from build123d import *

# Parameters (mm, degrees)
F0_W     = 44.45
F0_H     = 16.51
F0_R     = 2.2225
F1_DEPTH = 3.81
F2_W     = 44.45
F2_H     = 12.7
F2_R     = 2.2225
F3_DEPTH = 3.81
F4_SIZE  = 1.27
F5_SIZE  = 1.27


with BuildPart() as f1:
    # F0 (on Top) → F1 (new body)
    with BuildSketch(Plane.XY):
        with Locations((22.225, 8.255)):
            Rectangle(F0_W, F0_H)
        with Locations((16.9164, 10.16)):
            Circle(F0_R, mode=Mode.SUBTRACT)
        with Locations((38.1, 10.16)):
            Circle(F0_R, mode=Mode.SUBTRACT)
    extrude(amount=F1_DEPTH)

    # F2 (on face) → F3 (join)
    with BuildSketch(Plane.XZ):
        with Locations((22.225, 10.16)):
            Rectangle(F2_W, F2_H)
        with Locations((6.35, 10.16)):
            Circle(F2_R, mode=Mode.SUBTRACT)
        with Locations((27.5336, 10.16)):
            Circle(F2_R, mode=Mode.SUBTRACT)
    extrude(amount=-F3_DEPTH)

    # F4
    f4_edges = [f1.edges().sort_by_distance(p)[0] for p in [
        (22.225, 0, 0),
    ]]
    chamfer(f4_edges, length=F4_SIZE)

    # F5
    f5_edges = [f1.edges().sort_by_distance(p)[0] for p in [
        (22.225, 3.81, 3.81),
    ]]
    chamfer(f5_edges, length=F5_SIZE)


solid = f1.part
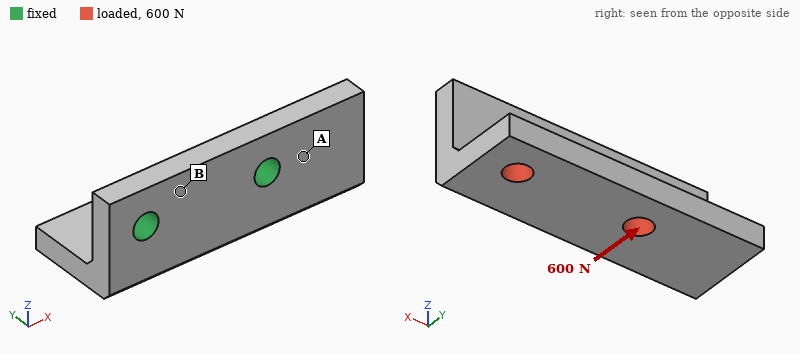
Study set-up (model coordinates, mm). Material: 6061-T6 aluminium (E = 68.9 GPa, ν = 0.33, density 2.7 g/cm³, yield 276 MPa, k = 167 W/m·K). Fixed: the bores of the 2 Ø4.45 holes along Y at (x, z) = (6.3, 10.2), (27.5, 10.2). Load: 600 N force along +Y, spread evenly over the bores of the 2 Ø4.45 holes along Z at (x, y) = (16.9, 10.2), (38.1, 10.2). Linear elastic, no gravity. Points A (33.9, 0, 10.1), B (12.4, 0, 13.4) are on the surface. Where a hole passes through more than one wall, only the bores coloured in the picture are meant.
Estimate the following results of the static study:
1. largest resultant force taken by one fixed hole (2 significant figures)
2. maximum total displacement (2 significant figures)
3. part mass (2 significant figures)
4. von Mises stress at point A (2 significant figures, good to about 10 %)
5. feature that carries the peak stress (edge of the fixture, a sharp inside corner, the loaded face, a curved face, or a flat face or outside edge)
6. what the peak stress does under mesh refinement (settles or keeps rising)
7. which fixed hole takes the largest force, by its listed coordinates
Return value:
550 N
46 µm
13 g
25 MPa
edge of the fixture
keeps rising
(27.5, 10.2)
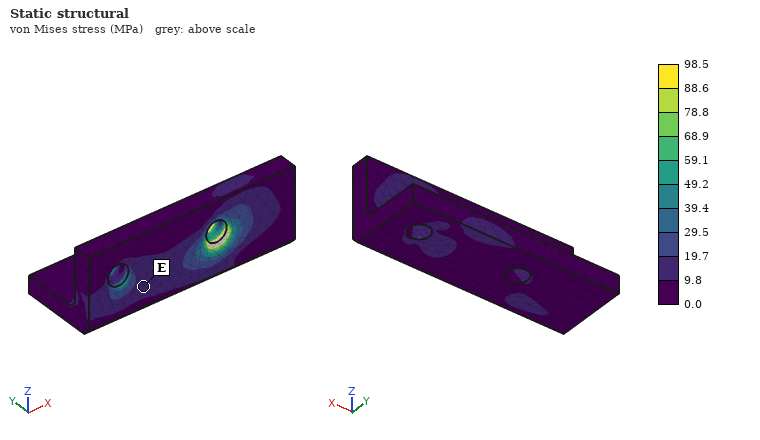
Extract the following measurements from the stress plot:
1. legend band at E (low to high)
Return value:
9.8 to 19.7 MPa
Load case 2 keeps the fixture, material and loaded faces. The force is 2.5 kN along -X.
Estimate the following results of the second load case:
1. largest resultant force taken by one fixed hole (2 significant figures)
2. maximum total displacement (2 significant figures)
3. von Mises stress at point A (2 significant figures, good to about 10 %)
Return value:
1.7 kN
73 µm
44 MPa
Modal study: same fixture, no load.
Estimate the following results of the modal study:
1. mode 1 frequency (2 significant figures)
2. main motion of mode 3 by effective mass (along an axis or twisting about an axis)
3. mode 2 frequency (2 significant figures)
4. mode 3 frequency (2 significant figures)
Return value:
7800 Hz
along Y
11 kHz
15 kHz
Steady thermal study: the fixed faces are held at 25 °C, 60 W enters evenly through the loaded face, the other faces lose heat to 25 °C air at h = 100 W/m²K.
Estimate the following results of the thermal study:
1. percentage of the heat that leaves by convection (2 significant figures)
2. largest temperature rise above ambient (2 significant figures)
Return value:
9.6 %
52 K
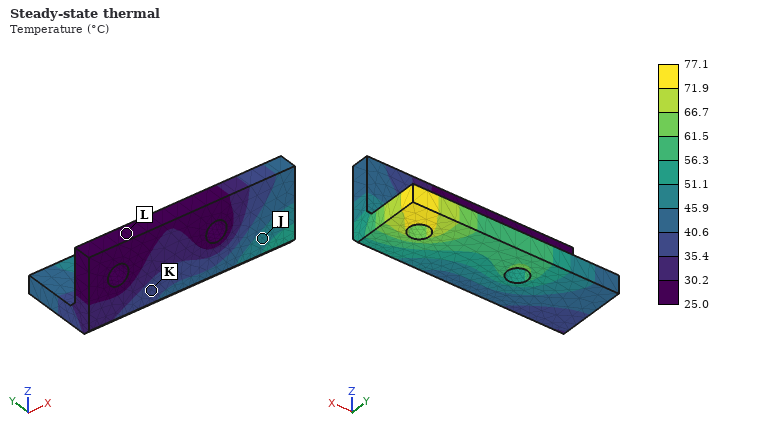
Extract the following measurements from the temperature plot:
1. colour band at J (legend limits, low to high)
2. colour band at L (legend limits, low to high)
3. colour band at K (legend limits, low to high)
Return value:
45.9 to 51.1 °C
25.0 to 30.2 °C
35.4 to 40.6 °C
